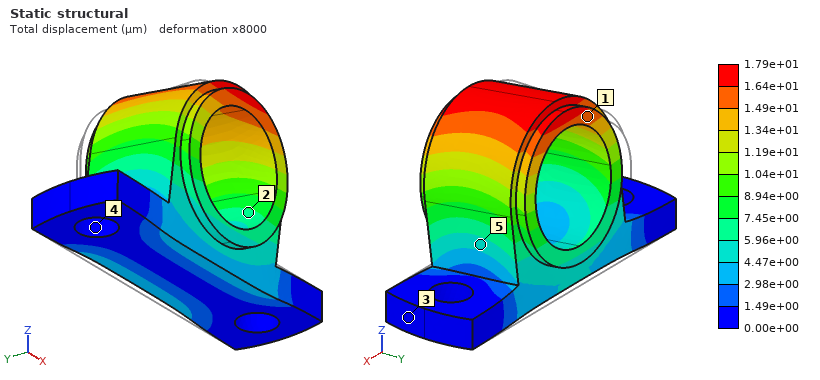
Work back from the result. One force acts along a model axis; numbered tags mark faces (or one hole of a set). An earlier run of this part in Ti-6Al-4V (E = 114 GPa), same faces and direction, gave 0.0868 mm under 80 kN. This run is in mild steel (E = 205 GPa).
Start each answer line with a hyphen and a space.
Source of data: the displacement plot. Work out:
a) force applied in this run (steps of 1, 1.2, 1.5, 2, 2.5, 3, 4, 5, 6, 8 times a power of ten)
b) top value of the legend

- 30 kN
- 1.79e+01 µm
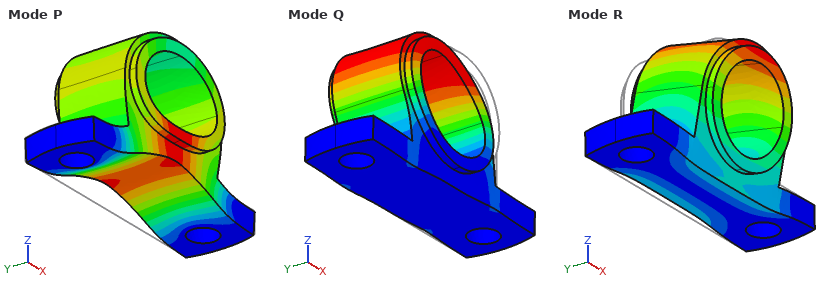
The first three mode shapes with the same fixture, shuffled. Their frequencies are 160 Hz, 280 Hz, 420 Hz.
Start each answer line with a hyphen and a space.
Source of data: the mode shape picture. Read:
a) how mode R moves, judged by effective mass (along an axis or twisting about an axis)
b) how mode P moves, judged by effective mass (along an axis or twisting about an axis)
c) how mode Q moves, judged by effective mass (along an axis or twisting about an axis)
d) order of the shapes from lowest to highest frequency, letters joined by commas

- along Y
- along Z
- along X
- R, Q, P
